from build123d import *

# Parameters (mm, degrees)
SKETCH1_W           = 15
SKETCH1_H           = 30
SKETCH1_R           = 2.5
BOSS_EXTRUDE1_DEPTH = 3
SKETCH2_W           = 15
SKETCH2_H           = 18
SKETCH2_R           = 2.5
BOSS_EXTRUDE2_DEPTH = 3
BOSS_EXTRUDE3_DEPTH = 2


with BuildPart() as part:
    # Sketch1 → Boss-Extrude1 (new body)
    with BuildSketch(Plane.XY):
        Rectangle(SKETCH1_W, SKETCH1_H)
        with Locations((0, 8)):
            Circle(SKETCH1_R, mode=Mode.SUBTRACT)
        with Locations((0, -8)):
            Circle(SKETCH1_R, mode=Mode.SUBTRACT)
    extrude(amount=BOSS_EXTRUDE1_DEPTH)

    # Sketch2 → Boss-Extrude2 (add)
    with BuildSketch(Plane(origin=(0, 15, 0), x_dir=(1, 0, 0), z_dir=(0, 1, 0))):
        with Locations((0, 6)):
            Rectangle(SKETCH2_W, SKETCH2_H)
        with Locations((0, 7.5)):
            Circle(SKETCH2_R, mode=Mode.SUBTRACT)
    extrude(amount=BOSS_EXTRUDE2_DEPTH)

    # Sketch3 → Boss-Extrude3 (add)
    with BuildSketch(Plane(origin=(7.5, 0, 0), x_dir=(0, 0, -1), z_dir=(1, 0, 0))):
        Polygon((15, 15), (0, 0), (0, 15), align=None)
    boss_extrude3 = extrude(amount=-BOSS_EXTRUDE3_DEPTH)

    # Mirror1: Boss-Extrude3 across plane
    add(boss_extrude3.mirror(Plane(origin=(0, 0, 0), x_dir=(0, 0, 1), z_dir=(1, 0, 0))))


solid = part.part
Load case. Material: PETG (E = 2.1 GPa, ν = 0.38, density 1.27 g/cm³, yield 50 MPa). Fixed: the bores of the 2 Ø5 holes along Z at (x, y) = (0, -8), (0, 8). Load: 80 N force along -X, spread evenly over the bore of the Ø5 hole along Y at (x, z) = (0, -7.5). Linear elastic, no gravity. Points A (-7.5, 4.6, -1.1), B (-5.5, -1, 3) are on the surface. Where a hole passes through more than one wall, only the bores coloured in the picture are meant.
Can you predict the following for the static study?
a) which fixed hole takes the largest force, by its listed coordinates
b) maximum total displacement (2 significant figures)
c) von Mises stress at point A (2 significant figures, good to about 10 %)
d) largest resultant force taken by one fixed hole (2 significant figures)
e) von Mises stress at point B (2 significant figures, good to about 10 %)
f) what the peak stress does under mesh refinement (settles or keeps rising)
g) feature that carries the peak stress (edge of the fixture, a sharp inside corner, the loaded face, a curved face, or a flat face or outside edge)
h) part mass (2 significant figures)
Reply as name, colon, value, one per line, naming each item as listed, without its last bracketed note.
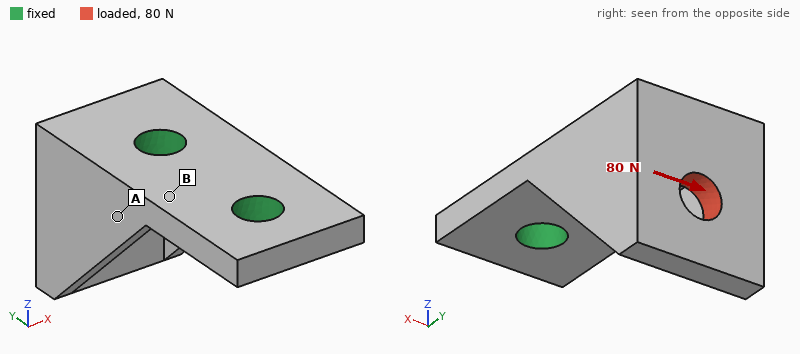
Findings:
which fixed hole takes the largest force, by its listed coordinates: (0, 8)
maximum total displacement: 0.42 mm
von Mises stress at point A: 6.8 MPa
largest resultant force taken by one fixed hole: 99 N
von Mises stress at point B: 3.0 MPa
what the peak stress does under mesh refinement: keeps rising
feature that carries the peak stress: edge of the fixture
part mass: 3.1 g
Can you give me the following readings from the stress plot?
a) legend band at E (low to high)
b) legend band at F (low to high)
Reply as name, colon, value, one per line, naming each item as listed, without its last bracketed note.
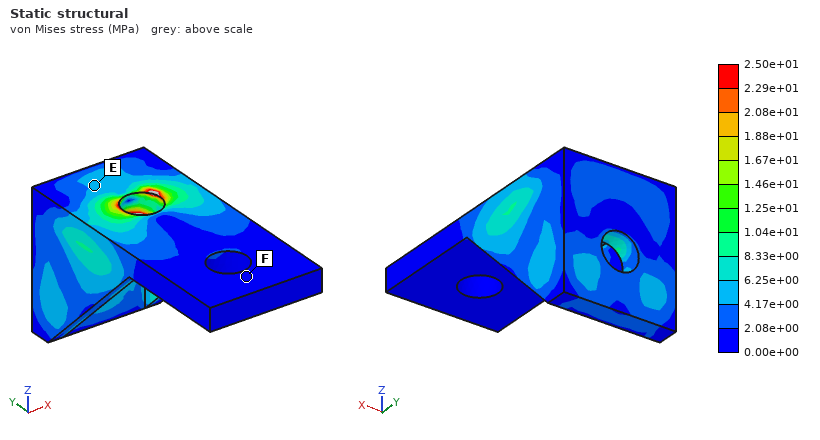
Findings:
legend band at E: 4.17e+00 to 6.25e+00 MPa
legend band at F: 0.00e+00 to 2.08e+00 MPa
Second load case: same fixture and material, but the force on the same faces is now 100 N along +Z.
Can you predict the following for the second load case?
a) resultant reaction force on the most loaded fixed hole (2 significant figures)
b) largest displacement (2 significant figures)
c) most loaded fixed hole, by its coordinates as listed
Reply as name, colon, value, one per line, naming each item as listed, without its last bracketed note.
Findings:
resultant reaction force on the most loaded fixed hole: 120 N
largest displacement: 0.21 mm
most loaded fixed hole, by its coordinates as listed: (0, 8)
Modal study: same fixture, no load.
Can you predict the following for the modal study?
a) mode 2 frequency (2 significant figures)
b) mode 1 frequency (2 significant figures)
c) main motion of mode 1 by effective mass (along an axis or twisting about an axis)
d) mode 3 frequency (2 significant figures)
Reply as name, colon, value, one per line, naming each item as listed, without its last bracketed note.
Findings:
mode 2 frequency: 3200 Hz
mode 1 frequency: 2400 Hz
main motion of mode 1 by effective mass: along X
mode 3 frequency: 6600 Hz
